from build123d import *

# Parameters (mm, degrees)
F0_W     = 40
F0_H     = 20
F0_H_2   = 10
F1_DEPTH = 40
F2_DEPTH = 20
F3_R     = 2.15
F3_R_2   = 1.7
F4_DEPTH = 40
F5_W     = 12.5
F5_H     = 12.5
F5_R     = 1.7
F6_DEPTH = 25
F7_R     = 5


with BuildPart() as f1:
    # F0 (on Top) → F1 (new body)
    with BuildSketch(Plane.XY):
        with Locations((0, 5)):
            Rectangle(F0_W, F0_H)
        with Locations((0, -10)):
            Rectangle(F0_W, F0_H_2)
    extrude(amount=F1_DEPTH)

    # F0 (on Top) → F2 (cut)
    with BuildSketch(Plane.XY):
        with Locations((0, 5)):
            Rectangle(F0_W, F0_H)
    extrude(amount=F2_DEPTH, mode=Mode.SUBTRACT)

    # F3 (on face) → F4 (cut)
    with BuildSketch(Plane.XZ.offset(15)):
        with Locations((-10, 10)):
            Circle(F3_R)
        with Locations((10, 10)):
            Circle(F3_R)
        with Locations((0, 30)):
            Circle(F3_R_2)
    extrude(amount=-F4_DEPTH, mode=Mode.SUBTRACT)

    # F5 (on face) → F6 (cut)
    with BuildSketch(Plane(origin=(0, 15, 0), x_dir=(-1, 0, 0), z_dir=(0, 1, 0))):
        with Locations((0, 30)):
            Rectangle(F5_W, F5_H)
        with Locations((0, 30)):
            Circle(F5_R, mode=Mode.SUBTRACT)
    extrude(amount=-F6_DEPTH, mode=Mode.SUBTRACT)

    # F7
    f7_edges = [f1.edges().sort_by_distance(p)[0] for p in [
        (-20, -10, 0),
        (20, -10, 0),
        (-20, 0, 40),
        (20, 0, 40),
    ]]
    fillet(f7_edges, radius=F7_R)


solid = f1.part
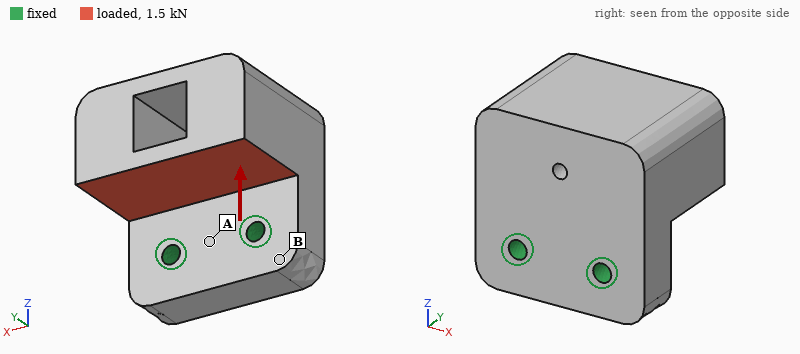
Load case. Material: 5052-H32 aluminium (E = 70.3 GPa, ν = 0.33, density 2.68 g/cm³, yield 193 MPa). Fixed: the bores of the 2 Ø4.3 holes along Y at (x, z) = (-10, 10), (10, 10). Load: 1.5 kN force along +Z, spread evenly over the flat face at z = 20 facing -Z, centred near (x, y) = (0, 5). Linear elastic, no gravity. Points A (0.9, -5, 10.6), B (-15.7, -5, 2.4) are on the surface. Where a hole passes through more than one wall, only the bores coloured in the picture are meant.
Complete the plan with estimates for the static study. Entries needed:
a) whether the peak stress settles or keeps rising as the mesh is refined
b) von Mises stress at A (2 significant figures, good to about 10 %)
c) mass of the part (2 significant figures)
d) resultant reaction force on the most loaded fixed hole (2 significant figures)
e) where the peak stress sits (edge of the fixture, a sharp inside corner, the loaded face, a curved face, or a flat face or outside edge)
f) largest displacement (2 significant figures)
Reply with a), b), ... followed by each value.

a) keeps rising
b) 15 MPa
c) 73 g
d) 750 N
e) edge of the fixture
f) 55 µm
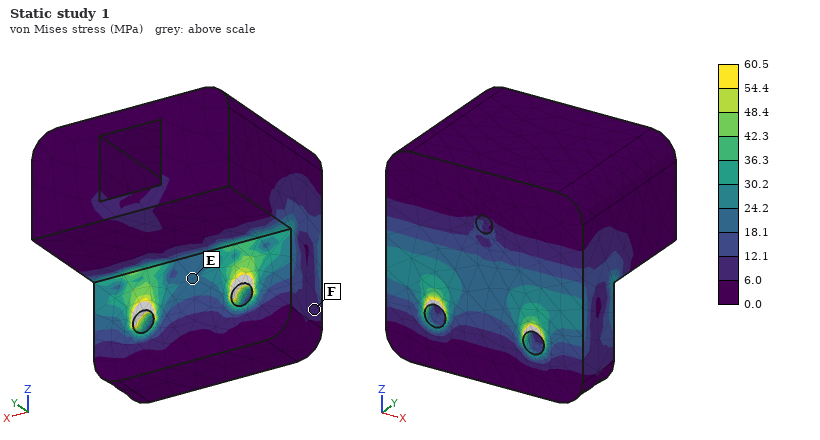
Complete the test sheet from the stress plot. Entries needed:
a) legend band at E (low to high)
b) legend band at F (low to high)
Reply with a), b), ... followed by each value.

a) 18.1 to 24.2 MPa
b) 6.0 to 12.1 MPa
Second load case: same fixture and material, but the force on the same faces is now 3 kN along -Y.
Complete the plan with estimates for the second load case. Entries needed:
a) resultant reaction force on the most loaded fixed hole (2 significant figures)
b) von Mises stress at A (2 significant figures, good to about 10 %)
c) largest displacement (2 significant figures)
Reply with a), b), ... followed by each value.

a) 1.5 kN
b) 15 MPa
c) 27 µm
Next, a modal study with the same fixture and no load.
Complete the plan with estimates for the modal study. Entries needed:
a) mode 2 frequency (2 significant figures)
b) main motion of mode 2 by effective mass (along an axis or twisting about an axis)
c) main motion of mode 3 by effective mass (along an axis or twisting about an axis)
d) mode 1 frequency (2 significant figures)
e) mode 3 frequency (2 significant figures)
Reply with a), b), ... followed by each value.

a) 7300 Hz
b) along X
c) along X
d) 4100 Hz
e) 11 kHz
